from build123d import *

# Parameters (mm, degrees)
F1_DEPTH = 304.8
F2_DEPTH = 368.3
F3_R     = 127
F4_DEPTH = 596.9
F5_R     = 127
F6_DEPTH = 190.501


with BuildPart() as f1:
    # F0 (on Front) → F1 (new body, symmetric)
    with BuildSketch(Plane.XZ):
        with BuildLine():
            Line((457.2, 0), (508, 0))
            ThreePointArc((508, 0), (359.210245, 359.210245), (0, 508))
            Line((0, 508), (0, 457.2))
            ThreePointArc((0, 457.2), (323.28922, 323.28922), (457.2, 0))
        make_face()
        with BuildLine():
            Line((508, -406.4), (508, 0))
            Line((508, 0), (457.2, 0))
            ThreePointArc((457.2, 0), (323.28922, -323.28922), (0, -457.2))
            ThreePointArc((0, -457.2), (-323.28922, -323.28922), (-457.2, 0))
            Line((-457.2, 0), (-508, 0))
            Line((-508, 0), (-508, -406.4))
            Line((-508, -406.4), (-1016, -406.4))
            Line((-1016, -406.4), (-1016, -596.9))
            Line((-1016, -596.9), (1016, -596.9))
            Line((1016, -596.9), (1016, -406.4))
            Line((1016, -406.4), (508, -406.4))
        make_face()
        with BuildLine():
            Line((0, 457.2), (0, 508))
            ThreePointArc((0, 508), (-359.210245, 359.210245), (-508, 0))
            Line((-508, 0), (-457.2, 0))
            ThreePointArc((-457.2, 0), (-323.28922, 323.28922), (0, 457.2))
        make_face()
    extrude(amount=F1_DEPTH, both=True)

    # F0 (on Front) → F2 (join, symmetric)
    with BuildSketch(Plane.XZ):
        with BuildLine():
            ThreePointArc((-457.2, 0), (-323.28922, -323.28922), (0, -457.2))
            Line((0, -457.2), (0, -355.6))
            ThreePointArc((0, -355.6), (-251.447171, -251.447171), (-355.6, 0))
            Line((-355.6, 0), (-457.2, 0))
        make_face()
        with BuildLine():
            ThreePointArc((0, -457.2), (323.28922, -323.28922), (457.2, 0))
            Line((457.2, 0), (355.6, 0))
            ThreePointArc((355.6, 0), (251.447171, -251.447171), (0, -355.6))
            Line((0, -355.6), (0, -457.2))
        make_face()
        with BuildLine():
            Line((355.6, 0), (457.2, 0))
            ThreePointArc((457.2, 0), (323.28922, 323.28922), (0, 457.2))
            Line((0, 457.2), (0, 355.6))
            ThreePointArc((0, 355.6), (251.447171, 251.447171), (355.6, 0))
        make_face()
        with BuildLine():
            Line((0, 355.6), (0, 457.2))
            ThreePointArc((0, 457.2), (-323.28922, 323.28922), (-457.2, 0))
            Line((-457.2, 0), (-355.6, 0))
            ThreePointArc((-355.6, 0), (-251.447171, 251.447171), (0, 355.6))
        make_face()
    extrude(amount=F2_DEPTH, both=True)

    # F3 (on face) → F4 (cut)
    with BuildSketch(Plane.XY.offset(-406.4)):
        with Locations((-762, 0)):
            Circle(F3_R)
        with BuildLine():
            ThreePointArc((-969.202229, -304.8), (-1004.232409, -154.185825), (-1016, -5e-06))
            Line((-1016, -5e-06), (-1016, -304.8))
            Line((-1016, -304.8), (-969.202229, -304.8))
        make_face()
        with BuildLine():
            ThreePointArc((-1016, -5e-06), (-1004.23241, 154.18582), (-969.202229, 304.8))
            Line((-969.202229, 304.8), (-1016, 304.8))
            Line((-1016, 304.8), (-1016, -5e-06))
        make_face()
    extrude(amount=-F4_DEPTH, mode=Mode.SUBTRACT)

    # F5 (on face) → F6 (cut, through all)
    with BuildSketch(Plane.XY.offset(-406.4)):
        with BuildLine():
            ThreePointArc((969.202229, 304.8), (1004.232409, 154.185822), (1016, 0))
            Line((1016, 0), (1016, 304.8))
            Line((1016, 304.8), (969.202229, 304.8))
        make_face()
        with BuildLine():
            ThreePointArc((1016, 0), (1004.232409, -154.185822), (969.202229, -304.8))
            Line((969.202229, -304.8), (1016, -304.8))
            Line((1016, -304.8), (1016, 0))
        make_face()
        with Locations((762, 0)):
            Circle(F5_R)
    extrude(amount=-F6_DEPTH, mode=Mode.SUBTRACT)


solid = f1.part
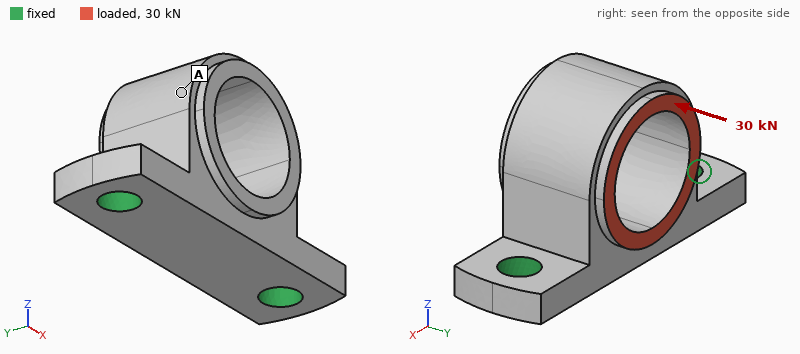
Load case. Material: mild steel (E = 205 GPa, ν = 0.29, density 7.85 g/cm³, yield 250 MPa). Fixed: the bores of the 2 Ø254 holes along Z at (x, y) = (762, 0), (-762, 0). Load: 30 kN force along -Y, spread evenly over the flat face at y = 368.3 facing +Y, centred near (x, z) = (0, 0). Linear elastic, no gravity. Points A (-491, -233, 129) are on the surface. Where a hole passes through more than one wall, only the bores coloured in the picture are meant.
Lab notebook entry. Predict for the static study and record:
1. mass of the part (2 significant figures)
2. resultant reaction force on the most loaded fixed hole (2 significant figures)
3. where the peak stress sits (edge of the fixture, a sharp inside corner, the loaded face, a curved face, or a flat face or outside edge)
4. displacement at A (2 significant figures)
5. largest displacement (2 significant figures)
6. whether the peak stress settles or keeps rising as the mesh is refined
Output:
3900 kg
15 kN
edge of the fixture
11 µm
18 µm
keeps rising
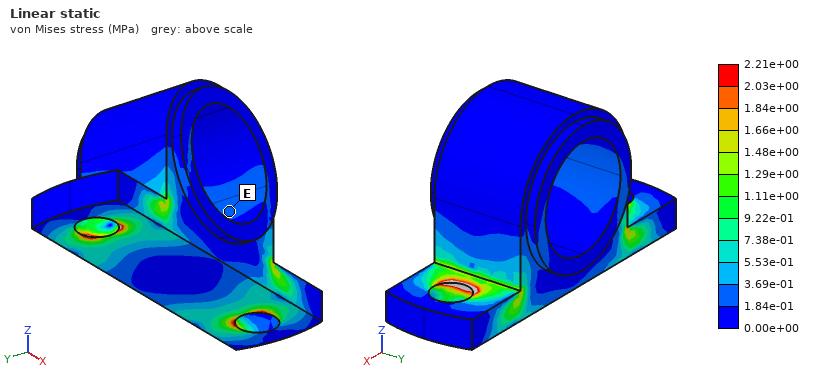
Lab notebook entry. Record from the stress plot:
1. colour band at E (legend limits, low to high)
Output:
1.84e-01 to 3.69e-01 MPa
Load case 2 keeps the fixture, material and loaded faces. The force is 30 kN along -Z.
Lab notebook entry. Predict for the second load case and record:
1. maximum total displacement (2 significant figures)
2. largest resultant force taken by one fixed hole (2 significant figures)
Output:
14 µm
16 kN
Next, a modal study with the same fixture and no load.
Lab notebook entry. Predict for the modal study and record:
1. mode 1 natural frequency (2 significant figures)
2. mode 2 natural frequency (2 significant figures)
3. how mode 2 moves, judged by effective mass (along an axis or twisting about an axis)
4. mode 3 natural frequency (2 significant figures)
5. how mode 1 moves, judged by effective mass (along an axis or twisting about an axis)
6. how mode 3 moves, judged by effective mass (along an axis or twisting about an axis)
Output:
160 Hz
280 Hz
along X
420 Hz
along Y
along Z
